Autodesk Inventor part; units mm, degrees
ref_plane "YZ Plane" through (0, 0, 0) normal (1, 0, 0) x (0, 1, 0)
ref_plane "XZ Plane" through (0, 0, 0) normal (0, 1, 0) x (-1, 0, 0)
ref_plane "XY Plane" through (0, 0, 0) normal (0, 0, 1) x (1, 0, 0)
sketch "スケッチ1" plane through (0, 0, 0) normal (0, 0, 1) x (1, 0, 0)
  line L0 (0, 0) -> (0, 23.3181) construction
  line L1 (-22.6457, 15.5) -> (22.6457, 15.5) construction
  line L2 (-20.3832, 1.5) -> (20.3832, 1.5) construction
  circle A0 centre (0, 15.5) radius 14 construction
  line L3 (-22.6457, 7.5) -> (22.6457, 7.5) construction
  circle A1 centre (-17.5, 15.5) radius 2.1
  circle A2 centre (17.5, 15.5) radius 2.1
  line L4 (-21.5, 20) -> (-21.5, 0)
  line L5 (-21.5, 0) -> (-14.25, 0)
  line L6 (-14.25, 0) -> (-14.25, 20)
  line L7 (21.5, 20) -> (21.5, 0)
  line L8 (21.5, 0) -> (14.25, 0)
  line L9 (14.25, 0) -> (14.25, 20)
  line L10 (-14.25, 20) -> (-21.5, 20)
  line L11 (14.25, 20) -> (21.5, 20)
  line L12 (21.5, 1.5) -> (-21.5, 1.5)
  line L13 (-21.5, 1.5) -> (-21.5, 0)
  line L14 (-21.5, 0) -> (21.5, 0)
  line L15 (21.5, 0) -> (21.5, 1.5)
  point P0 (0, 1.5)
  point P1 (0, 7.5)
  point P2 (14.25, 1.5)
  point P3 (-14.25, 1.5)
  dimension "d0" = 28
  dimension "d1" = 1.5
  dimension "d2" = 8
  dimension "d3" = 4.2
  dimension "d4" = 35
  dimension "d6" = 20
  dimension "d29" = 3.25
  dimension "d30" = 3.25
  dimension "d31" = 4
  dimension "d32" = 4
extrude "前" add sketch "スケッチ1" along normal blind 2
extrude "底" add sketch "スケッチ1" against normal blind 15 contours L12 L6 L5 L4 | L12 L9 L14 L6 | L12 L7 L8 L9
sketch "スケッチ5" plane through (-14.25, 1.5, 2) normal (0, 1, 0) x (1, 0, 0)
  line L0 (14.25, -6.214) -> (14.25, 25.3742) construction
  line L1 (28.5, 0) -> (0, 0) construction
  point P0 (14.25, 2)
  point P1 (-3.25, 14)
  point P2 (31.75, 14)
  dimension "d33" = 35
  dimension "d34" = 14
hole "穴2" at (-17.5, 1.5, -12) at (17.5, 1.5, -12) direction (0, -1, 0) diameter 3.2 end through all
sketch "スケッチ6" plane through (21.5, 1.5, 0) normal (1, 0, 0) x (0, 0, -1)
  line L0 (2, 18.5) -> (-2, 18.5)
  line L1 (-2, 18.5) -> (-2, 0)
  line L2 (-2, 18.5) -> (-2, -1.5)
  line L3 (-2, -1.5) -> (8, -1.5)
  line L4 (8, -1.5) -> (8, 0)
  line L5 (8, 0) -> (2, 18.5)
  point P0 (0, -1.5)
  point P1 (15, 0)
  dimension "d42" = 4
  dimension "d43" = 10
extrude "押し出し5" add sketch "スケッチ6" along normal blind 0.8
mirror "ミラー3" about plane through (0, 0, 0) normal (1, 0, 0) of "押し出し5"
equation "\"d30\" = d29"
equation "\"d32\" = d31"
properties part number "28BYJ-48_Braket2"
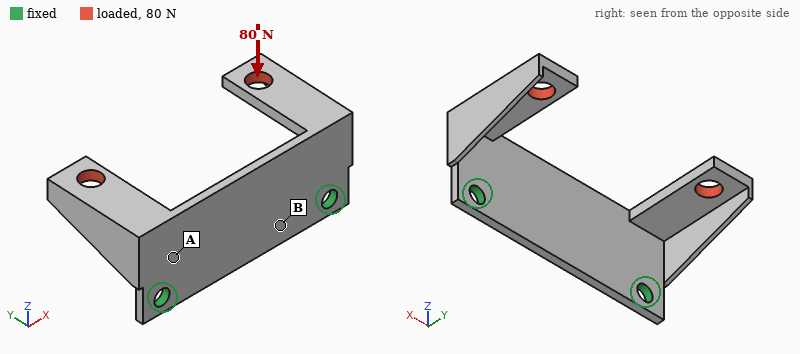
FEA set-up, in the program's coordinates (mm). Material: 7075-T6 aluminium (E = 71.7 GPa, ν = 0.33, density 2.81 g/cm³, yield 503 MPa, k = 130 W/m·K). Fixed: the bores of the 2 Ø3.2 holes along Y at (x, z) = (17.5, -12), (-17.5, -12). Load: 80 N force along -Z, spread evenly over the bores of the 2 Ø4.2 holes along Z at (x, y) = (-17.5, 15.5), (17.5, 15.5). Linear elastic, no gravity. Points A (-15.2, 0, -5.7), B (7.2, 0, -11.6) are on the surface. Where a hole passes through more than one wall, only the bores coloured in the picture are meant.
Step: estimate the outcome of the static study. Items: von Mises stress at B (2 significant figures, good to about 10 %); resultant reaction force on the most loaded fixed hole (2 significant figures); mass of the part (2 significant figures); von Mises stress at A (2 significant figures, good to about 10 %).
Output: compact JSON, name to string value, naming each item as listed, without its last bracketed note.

{"von Mises stress at B": "25 MPa", "resultant reaction force on the most loaded fixed hole": "40 N", "mass of the part": "5.0 g", "von Mises stress at A": "70 MPa"}
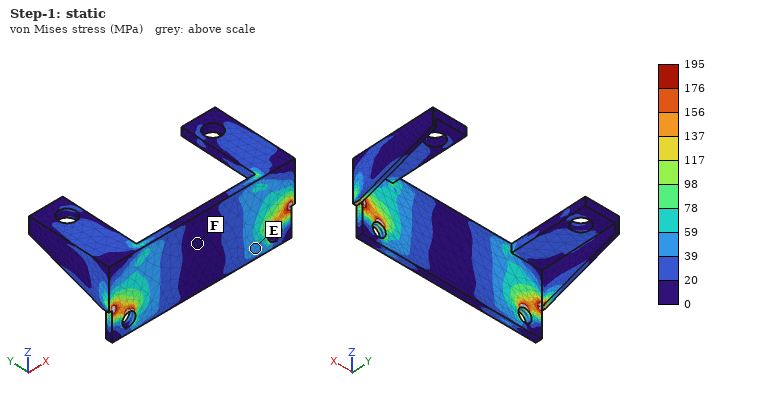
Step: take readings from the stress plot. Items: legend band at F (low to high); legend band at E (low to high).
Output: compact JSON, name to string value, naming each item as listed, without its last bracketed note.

{"legend band at F": "0 to 20 MPa", "legend band at E": "39 to 59 MPa"}
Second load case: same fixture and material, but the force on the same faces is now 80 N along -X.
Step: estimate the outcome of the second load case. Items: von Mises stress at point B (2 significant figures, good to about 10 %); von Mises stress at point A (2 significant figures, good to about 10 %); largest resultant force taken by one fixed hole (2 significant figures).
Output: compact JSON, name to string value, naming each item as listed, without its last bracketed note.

{"von Mises stress at point B": "14 MPa", "von Mises stress at point A": "56 MPa", "largest resultant force taken by one fixed hole": "51 N"}
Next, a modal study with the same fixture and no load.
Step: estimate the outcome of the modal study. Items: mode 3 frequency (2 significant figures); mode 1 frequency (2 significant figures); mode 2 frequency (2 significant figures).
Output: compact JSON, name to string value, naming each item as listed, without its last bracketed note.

{"mode 3 frequency": "2800 Hz", "mode 1 frequency": "2100 Hz", "mode 2 frequency": "2200 Hz"}
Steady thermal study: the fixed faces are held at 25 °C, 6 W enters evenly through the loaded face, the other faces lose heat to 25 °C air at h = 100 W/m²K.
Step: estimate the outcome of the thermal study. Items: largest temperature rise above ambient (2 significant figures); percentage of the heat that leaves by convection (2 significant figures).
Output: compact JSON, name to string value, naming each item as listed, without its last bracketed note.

{"largest temperature rise above ambient": "26 K", "percentage of the heat that leaves by convection": "40 %"}
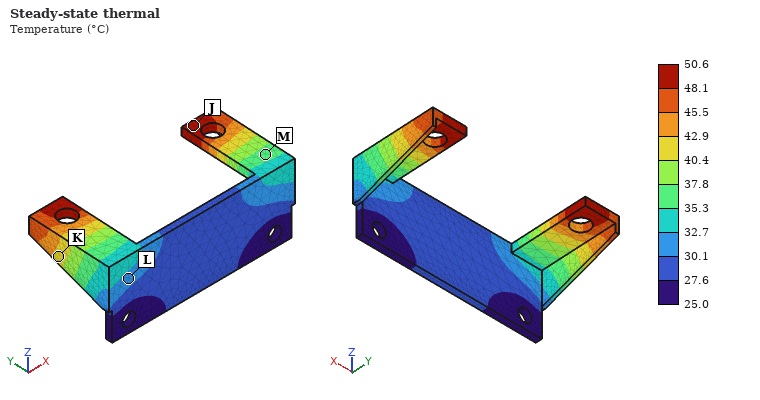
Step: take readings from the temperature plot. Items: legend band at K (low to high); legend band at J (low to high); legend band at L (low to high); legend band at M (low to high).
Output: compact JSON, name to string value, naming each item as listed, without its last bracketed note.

{"legend band at K": "40.4 to 42.9 °C", "legend band at J": "48.1 to 50.6 °C", "legend band at L": "30.1 to 32.7 °C", "legend band at M": "35.3 to 37.8 °C"}
